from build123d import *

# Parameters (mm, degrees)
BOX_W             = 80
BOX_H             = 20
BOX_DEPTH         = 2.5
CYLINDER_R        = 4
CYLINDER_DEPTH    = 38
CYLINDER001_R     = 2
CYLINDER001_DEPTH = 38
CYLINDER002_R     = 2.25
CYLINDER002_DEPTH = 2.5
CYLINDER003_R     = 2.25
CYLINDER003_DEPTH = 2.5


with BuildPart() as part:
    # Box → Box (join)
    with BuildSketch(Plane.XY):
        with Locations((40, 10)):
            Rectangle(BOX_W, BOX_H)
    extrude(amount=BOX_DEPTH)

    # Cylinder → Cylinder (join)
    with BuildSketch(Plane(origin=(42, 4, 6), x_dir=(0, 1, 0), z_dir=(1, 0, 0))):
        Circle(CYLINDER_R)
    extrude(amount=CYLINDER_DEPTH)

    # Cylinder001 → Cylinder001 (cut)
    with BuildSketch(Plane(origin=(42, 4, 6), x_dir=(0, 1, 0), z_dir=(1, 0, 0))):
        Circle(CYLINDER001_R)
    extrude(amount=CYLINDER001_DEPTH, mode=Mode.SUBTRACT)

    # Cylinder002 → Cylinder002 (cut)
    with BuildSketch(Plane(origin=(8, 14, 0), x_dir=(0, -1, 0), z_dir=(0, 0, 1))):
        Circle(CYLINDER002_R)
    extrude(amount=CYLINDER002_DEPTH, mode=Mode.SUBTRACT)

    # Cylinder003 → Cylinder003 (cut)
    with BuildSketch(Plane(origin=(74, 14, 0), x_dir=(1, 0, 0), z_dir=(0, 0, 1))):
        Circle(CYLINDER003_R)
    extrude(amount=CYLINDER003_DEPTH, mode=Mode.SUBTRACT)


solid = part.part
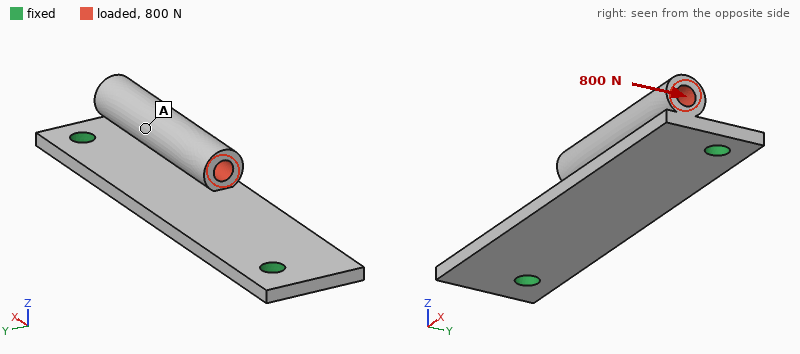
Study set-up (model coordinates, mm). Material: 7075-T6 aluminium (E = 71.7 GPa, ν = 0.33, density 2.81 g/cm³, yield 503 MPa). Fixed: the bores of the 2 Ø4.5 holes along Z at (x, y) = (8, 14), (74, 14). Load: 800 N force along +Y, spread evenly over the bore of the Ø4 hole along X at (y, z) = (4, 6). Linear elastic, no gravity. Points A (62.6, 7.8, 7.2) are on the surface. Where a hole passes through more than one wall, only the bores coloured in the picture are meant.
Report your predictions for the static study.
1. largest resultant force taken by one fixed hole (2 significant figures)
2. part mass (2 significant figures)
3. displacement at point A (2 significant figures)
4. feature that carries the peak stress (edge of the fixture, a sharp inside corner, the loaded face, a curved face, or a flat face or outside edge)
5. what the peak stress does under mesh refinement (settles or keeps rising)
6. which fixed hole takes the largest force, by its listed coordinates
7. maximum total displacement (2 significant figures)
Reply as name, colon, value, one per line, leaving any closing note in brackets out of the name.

largest resultant force taken by one fixed hole: 670 N
part mass: 15 g
displacement at point A: 0.088 mm
feature that carries the peak stress: edge of the fixture
what the peak stress does under mesh refinement: keeps rising
which fixed hole takes the largest force, by its listed coordinates: (74, 14)
maximum total displacement: 0.16 mm
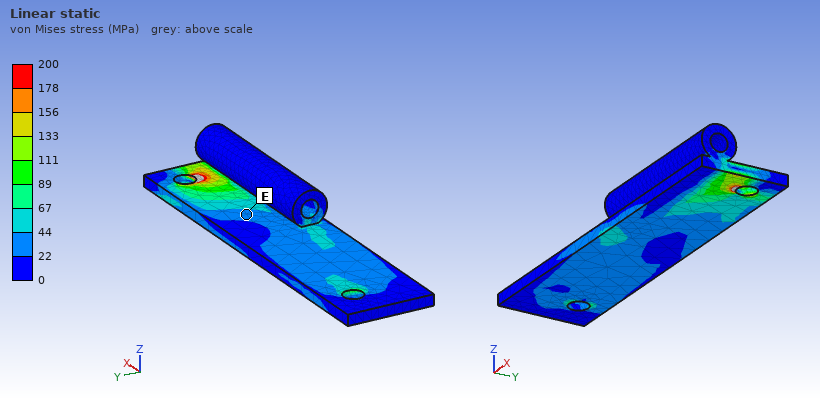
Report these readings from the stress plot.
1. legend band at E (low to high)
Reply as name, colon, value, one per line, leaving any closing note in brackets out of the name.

legend band at E: 22 to 44 MPa
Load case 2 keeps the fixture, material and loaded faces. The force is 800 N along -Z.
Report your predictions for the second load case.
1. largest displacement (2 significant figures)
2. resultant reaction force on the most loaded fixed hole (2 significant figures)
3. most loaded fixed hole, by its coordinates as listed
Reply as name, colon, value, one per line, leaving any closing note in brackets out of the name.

largest displacement: 0.40 mm
resultant reaction force on the most loaded fixed hole: 660 N
most loaded fixed hole, by its coordinates as listed: (74, 14)
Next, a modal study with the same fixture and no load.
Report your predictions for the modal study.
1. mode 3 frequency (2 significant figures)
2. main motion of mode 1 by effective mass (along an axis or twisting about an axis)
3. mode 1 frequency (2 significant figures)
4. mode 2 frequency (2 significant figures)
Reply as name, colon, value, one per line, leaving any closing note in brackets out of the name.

mode 3 frequency: 8800 Hz
main motion of mode 1 by effective mass: along Z
mode 1 frequency: 2700 Hz
mode 2 frequency: 4700 Hz
